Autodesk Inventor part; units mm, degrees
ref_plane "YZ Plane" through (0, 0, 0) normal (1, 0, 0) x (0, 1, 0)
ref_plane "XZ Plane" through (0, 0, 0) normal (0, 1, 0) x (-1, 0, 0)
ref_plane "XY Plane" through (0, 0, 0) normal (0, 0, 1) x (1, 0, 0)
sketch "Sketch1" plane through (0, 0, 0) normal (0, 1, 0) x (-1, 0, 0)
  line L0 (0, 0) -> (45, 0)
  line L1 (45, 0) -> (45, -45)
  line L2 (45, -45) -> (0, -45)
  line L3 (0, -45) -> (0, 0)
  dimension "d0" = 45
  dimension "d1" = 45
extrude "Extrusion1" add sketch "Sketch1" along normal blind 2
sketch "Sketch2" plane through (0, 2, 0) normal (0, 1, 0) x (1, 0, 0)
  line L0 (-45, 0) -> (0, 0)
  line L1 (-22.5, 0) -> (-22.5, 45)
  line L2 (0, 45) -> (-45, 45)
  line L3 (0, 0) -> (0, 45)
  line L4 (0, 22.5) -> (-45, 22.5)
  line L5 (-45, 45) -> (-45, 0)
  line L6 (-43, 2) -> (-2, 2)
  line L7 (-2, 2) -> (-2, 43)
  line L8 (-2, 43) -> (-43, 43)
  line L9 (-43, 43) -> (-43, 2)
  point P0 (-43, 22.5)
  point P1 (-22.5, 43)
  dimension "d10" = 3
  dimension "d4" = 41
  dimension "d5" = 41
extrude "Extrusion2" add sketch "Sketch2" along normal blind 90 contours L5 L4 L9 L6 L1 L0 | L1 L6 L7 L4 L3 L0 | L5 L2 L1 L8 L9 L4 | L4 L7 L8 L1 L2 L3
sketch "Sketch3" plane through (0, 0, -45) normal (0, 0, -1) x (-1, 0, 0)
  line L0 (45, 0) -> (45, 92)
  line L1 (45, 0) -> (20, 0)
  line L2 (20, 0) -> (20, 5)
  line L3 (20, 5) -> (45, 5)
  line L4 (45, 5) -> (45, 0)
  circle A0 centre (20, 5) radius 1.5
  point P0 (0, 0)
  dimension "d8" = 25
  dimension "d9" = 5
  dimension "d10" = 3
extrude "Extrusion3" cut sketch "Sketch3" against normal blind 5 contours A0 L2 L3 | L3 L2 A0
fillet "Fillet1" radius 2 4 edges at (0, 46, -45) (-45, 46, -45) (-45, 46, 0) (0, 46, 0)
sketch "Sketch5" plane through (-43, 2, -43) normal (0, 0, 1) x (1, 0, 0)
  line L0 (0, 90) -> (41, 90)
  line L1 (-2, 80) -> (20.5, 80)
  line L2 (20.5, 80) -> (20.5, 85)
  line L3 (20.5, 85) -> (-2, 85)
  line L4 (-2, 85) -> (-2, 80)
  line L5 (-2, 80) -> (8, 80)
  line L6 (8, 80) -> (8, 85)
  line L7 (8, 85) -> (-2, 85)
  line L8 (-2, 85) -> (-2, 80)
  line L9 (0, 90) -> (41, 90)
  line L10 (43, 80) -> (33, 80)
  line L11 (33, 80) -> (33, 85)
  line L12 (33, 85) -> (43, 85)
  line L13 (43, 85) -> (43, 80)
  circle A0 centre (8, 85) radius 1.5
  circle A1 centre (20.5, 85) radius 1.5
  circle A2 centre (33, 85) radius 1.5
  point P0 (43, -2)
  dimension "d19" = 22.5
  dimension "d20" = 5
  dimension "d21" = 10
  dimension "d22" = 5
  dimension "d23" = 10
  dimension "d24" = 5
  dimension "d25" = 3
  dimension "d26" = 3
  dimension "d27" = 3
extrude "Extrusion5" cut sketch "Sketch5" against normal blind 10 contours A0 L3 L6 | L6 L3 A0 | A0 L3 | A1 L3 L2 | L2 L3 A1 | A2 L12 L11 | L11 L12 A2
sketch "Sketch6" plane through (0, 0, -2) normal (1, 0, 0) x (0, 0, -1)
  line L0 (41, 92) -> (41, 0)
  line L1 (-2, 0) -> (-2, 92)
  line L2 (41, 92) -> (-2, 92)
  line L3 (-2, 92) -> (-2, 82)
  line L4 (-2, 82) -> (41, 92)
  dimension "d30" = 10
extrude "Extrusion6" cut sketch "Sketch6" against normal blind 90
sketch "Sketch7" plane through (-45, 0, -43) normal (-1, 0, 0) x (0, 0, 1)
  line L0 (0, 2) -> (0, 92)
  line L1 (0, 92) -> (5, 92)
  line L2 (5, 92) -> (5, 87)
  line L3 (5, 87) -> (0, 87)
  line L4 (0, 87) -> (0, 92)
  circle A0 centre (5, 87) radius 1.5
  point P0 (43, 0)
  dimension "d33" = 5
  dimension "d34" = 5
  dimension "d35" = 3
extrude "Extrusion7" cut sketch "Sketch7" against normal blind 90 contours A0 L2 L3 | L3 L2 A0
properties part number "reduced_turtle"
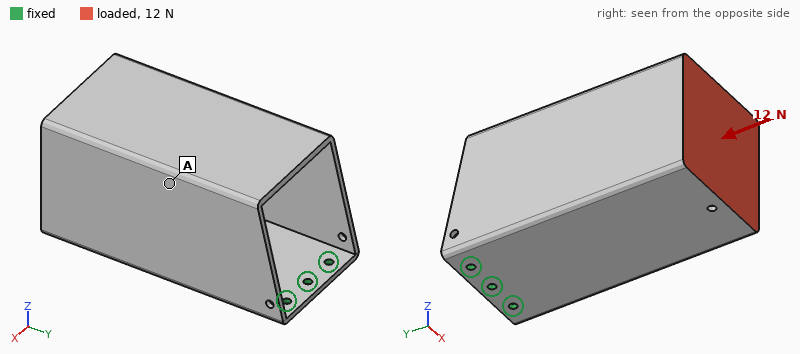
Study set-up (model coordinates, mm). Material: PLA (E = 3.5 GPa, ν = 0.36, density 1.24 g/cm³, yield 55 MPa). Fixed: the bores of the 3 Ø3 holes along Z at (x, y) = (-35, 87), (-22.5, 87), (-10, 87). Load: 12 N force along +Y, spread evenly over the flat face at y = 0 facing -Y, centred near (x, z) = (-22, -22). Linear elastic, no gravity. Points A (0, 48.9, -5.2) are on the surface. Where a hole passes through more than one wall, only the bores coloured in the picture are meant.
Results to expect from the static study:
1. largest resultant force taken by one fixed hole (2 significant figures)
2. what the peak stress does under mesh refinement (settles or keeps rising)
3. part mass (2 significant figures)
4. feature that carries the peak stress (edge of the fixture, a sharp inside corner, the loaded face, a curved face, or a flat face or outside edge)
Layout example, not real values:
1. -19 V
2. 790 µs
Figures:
1. 5.9 N
2. keeps rising
3. 41 g
4. edge of the fixture
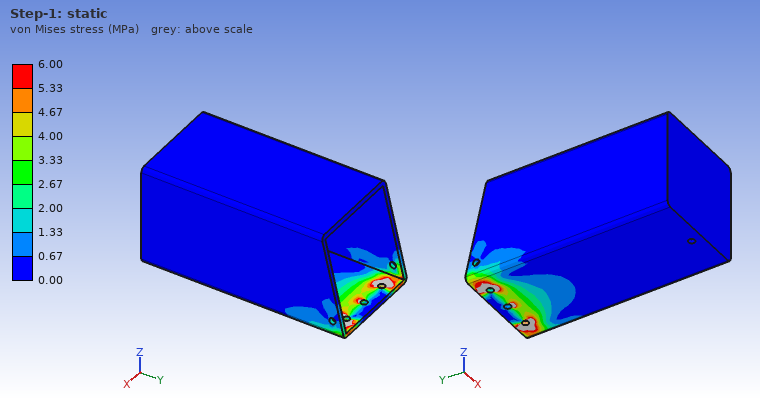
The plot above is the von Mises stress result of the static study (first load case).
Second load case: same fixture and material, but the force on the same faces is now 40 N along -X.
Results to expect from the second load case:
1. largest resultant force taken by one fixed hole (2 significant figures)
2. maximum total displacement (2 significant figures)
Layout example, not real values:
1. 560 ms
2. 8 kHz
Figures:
1. 130 N
2. 1.1 mm
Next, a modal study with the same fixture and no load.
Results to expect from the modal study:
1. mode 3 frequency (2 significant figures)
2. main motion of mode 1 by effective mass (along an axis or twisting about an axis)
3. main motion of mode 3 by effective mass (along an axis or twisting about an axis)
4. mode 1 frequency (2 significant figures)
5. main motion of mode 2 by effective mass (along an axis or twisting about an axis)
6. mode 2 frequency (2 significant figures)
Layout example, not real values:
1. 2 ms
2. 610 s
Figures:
1. 620 Hz
2. along Z
3. along X
4. 60 Hz
5. along X
6. 150 Hz
